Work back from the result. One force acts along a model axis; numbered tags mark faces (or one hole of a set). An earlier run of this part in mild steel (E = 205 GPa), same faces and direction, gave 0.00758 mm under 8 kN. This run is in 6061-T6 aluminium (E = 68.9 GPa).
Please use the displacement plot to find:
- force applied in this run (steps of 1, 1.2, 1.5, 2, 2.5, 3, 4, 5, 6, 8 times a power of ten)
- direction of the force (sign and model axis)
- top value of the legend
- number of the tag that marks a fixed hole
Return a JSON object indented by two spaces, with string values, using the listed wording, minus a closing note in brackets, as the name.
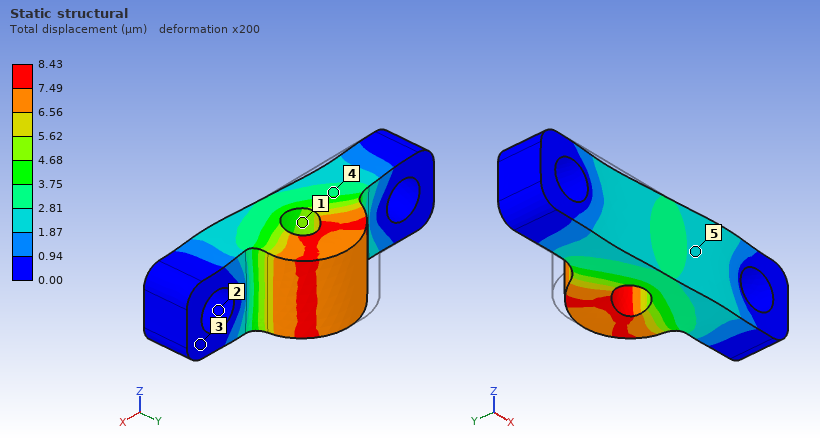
{
  "force applied in this run": "3 kN",
  "direction of the force": "+X",
  "top value of the legend": "8.43 µm",
  "number of the tag that marks a fixed hole": "2"
}
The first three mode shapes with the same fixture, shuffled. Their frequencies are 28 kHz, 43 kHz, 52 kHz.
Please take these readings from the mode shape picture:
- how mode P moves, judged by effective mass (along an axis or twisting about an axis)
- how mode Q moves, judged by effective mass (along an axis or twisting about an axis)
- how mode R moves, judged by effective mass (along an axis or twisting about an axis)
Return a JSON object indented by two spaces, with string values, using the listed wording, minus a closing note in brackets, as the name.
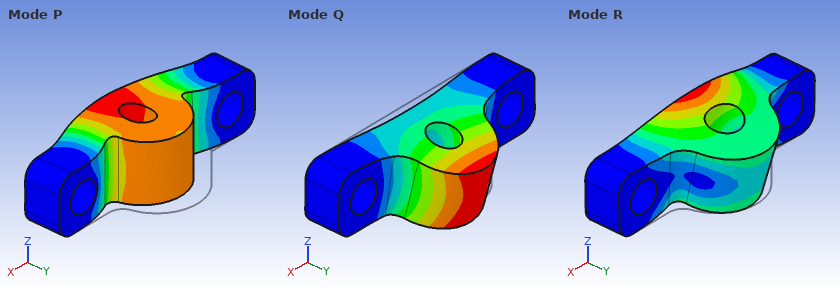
{
  "how mode P moves, judged by effective mass": "along Y",
  "how mode Q moves, judged by effective mass": "along Z",
  "how mode R moves, judged by effective mass": "along Z"
}
